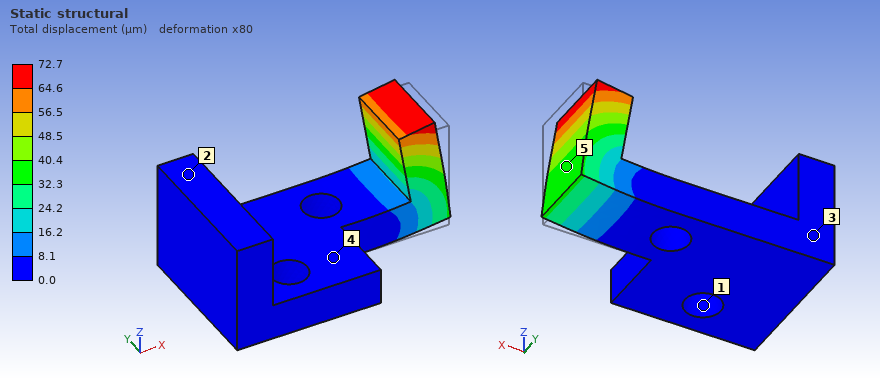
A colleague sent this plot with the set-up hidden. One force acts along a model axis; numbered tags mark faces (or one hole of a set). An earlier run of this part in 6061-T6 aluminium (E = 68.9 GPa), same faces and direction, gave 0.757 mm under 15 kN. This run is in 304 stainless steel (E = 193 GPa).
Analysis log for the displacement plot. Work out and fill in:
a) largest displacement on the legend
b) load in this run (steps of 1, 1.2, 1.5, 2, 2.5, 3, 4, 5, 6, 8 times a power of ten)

72.7 µm
4 kN
